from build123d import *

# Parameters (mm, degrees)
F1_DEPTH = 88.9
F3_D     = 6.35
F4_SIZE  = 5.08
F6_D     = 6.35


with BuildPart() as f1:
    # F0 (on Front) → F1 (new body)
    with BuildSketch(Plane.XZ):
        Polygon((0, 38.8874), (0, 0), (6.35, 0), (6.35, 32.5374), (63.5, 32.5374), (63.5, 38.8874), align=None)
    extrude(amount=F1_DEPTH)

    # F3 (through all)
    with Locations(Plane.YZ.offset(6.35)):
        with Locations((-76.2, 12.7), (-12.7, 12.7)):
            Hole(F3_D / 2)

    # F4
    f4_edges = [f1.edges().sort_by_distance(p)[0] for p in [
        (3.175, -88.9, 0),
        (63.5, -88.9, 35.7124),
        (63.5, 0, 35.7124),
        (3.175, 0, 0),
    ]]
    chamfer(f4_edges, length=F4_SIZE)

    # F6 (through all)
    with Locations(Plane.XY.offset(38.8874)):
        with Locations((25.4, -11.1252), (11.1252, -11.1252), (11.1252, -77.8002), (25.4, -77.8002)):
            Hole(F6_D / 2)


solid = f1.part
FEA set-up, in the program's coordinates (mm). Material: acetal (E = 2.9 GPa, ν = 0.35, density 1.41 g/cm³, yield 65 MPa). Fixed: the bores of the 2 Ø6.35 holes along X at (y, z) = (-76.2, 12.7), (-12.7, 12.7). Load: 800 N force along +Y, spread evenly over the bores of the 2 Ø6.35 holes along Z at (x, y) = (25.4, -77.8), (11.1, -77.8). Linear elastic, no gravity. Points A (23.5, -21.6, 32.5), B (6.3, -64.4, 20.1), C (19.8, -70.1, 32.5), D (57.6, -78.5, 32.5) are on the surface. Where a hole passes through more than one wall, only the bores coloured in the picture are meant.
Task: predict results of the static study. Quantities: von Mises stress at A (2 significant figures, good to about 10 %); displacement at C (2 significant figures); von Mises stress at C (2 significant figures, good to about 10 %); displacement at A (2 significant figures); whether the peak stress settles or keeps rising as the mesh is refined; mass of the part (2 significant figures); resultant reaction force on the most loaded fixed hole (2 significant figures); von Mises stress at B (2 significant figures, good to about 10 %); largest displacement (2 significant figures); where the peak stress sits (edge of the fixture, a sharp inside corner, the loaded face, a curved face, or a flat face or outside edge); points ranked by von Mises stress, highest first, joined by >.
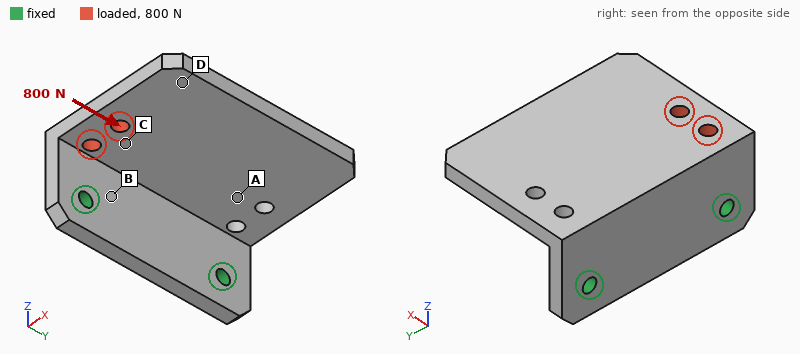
2.8 MPa
0.27 mm
4.9 MPa
0.26 mm
keeps rising
74 g
520 N
7.0 MPa
0.61 mm
edge of the fixture
B > C > A > D
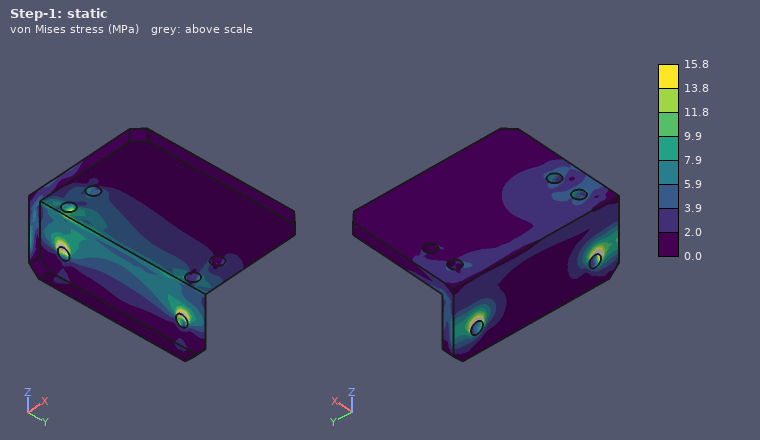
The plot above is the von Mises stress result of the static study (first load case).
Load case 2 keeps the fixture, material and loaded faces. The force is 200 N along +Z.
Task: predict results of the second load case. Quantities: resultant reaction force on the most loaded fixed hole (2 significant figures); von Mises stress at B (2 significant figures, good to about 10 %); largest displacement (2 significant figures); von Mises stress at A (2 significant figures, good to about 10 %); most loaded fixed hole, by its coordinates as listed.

200 N
5.5 MPa
1.4 mm
2.1 MPa
(-76.2, 12.7)
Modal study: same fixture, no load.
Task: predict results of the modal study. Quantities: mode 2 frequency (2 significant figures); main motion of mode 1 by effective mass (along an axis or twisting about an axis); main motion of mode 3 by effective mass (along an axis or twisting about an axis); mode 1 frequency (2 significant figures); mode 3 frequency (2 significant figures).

550 Hz
along Z
along Y
250 Hz
830 Hz
